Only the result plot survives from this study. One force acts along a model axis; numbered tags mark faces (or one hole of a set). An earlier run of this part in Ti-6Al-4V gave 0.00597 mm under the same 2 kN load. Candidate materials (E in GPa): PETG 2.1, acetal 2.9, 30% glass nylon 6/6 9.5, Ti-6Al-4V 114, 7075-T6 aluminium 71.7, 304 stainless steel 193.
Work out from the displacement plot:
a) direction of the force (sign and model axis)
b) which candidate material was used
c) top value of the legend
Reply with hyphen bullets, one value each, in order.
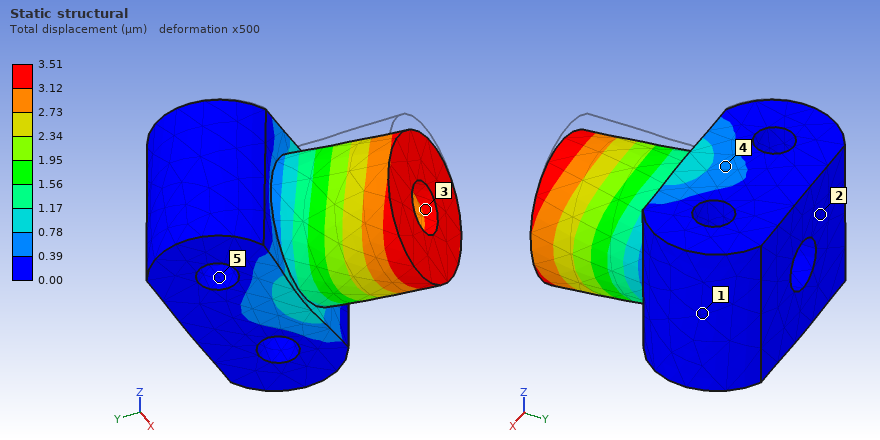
- -Z
- 304 stainless steel
- 3.51 µm
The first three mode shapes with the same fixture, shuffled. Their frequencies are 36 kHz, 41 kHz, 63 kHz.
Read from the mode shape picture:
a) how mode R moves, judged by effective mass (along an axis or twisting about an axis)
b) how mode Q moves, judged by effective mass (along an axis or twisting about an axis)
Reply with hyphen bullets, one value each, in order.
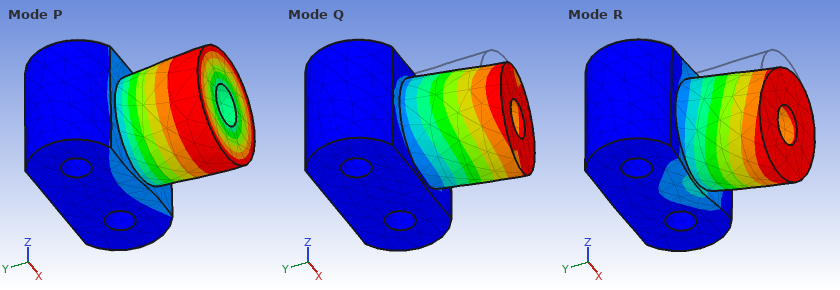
- along Z
- along X
